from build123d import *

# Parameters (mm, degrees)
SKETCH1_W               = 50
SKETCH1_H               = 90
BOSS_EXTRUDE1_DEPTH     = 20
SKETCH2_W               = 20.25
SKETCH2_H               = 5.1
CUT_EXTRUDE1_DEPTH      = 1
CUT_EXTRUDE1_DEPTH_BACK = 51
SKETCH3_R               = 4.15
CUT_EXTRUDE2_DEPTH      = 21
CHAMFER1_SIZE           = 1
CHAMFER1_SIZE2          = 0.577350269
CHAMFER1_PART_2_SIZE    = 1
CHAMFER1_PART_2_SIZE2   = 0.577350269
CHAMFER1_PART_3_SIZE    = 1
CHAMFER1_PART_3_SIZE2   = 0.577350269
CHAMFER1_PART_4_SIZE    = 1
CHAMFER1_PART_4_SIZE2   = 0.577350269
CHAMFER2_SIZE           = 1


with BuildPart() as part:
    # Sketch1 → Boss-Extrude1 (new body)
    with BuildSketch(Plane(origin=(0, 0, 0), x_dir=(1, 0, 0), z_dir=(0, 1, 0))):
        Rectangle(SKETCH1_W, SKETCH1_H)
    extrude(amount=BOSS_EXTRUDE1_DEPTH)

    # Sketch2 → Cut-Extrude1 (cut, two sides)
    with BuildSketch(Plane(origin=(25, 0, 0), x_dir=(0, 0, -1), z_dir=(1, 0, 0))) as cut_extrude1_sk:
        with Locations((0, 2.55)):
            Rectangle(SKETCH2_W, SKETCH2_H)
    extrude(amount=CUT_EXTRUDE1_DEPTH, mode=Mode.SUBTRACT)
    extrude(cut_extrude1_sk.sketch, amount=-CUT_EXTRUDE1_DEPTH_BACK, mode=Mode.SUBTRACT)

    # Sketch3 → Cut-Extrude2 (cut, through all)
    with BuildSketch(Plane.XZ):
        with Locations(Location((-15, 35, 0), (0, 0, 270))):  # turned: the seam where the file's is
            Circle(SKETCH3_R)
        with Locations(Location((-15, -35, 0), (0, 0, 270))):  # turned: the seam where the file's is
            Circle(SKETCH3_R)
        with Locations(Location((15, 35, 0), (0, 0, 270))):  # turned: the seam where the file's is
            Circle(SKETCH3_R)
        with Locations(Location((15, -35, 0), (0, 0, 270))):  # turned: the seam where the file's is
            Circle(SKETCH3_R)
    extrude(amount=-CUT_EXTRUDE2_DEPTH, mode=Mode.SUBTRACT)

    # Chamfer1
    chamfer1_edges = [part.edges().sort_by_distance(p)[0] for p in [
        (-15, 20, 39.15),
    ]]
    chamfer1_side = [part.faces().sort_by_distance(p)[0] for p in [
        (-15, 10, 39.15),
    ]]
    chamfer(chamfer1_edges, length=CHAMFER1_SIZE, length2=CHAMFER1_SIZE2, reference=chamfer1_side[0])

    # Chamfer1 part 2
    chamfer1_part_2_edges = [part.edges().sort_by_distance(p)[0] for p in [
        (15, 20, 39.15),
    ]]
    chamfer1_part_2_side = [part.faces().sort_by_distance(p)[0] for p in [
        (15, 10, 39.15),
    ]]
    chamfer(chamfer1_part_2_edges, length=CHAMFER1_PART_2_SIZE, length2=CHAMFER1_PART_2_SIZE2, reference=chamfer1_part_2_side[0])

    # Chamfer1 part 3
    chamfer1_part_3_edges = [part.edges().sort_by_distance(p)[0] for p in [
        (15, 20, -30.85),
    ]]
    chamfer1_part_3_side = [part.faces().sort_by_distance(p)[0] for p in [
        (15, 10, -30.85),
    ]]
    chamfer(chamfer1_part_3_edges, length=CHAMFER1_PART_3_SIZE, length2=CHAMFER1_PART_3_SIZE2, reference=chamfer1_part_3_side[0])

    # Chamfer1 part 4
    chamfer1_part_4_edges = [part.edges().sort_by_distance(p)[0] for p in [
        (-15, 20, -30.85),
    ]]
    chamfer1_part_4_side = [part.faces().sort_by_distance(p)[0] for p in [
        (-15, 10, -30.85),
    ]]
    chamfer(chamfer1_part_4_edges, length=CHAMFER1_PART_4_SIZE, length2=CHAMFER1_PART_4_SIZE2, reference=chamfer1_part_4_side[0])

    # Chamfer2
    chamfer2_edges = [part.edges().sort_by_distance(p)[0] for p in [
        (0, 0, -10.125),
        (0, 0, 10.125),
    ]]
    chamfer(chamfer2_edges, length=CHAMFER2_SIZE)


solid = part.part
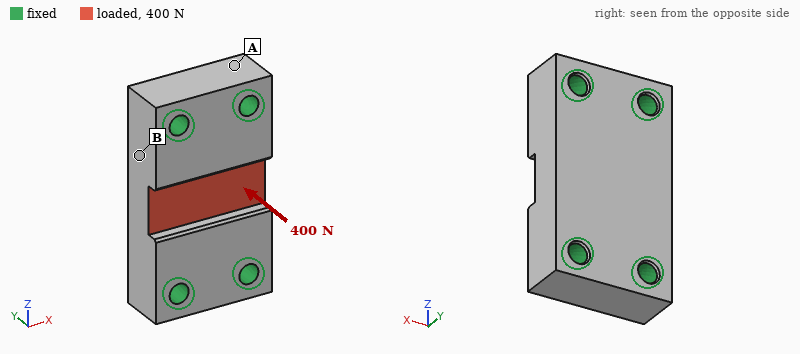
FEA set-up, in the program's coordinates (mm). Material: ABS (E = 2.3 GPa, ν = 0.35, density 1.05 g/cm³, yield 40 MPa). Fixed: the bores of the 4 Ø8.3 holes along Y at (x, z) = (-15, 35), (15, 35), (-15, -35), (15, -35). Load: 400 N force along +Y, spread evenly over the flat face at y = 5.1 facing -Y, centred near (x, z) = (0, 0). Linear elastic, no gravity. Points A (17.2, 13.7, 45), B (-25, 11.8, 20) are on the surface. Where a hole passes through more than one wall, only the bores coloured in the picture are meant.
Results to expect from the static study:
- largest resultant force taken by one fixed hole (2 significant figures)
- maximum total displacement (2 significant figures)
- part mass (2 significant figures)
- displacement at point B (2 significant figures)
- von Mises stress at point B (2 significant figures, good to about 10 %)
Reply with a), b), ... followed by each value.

a) 110 N
b) 22 µm
c) 84 g
d) 7.5 µm
e) 0.65 MPa
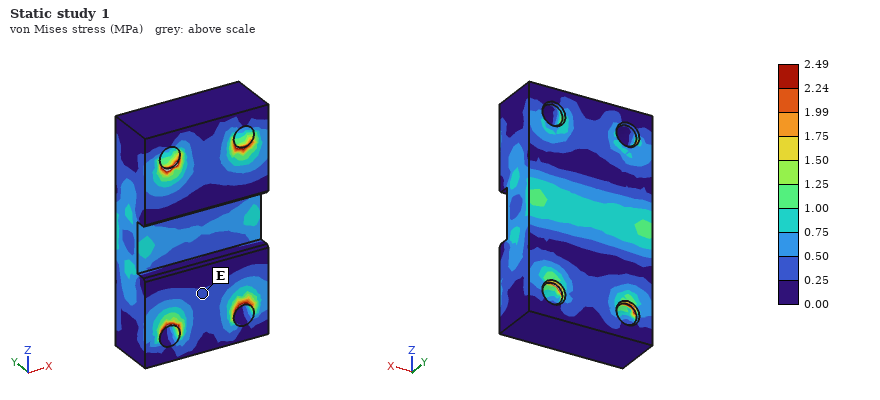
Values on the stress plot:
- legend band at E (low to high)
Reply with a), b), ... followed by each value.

a) 0.25 to 0.50 MPa
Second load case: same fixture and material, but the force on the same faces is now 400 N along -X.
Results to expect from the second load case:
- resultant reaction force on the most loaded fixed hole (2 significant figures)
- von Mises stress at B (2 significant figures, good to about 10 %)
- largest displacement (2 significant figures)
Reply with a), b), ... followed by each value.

a) 130 N
b) 0.31 MPa
c) 18 µm
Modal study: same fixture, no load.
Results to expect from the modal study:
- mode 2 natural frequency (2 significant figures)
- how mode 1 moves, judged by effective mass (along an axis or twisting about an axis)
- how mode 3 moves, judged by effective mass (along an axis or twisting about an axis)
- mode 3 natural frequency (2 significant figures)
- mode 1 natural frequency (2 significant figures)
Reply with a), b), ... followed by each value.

a) 5600 Hz
b) along Y
c) along X
d) 6200 Hz
e) 4400 Hz
